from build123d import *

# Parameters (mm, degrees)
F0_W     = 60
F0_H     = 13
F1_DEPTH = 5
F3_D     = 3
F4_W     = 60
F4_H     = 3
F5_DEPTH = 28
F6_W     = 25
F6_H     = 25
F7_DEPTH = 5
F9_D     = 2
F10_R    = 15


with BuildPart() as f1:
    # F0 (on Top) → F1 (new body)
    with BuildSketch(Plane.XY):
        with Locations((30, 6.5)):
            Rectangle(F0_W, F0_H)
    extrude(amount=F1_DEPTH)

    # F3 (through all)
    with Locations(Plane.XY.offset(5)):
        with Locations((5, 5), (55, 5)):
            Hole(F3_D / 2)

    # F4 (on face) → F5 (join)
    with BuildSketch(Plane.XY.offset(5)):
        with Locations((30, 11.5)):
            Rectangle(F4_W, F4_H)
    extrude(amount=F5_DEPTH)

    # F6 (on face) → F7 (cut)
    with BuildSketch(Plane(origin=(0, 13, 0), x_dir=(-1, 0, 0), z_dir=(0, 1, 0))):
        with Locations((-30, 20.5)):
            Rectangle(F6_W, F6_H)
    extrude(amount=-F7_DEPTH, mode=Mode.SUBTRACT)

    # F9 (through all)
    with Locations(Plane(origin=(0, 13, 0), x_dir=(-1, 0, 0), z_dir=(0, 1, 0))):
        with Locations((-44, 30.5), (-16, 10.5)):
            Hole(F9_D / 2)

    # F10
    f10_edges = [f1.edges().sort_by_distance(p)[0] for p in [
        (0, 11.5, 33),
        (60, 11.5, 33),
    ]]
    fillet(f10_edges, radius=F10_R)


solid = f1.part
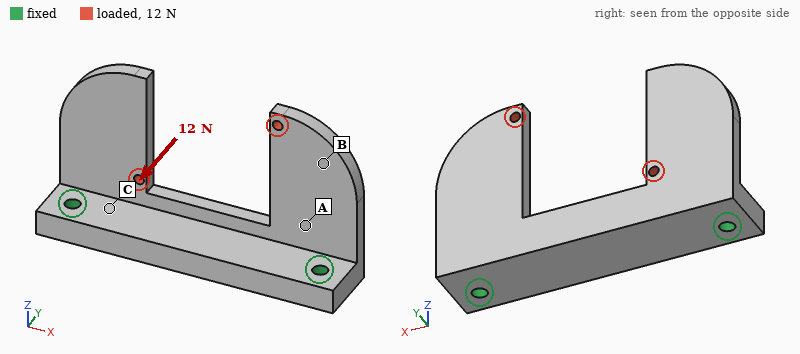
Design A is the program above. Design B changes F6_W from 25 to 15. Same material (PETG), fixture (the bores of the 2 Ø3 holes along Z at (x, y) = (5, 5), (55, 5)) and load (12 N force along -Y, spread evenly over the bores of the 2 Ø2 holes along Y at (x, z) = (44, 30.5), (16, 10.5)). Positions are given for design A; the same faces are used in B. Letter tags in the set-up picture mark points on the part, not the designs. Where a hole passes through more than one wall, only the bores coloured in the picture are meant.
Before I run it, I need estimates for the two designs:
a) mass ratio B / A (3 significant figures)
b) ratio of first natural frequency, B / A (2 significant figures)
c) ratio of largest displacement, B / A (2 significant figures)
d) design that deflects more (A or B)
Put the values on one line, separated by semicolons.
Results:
1.11; 0.93; 0.78; A
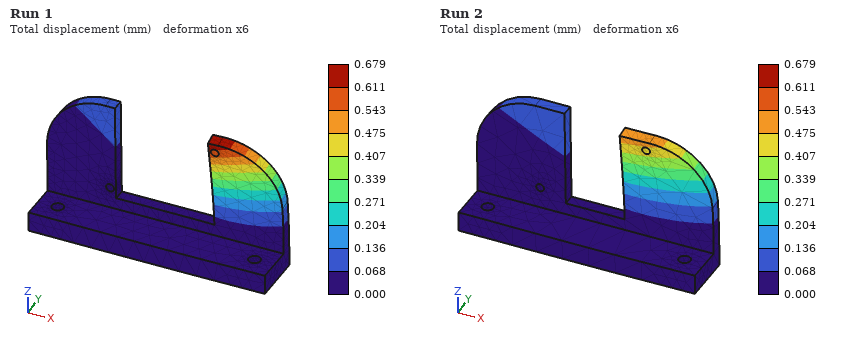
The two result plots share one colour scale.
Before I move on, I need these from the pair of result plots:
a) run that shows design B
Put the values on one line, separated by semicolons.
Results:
Run 2
